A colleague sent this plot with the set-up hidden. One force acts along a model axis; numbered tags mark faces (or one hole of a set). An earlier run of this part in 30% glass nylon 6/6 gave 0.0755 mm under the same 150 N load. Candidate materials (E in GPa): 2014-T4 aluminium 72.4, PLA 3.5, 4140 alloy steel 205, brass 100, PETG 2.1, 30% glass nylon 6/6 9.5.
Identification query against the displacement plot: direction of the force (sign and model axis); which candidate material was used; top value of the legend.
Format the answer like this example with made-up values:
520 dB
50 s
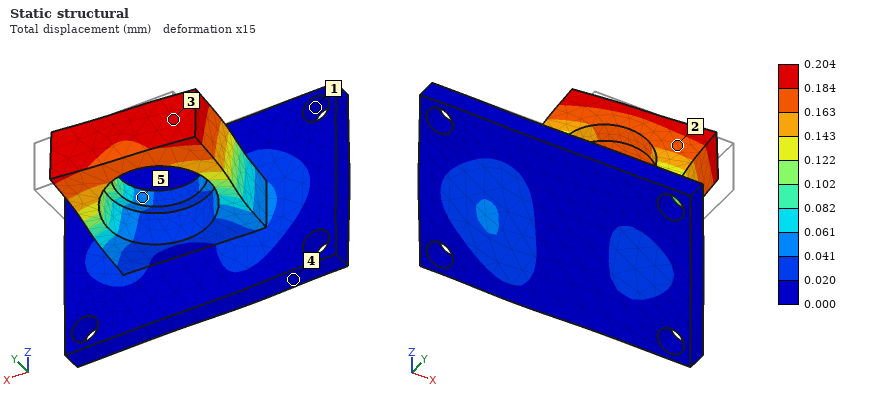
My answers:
-X
PLA
0.204 mm
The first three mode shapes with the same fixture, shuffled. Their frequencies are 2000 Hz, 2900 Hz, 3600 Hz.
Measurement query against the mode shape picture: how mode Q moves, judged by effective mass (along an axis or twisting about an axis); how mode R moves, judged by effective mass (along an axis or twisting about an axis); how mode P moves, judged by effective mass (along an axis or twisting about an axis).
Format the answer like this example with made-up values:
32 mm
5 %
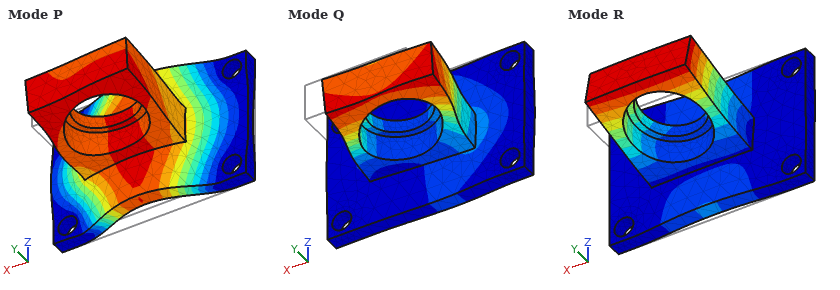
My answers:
along X
along Z
along Y
